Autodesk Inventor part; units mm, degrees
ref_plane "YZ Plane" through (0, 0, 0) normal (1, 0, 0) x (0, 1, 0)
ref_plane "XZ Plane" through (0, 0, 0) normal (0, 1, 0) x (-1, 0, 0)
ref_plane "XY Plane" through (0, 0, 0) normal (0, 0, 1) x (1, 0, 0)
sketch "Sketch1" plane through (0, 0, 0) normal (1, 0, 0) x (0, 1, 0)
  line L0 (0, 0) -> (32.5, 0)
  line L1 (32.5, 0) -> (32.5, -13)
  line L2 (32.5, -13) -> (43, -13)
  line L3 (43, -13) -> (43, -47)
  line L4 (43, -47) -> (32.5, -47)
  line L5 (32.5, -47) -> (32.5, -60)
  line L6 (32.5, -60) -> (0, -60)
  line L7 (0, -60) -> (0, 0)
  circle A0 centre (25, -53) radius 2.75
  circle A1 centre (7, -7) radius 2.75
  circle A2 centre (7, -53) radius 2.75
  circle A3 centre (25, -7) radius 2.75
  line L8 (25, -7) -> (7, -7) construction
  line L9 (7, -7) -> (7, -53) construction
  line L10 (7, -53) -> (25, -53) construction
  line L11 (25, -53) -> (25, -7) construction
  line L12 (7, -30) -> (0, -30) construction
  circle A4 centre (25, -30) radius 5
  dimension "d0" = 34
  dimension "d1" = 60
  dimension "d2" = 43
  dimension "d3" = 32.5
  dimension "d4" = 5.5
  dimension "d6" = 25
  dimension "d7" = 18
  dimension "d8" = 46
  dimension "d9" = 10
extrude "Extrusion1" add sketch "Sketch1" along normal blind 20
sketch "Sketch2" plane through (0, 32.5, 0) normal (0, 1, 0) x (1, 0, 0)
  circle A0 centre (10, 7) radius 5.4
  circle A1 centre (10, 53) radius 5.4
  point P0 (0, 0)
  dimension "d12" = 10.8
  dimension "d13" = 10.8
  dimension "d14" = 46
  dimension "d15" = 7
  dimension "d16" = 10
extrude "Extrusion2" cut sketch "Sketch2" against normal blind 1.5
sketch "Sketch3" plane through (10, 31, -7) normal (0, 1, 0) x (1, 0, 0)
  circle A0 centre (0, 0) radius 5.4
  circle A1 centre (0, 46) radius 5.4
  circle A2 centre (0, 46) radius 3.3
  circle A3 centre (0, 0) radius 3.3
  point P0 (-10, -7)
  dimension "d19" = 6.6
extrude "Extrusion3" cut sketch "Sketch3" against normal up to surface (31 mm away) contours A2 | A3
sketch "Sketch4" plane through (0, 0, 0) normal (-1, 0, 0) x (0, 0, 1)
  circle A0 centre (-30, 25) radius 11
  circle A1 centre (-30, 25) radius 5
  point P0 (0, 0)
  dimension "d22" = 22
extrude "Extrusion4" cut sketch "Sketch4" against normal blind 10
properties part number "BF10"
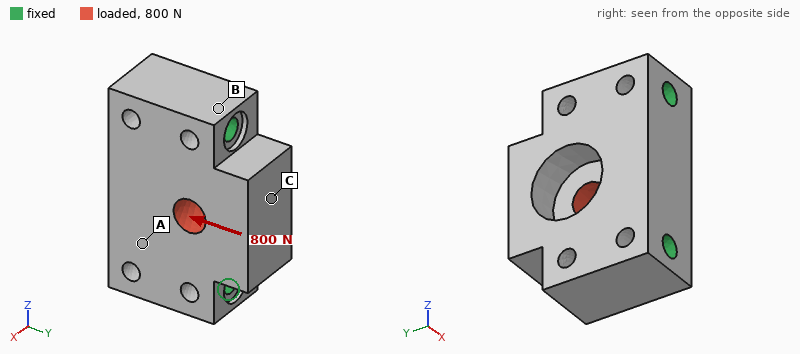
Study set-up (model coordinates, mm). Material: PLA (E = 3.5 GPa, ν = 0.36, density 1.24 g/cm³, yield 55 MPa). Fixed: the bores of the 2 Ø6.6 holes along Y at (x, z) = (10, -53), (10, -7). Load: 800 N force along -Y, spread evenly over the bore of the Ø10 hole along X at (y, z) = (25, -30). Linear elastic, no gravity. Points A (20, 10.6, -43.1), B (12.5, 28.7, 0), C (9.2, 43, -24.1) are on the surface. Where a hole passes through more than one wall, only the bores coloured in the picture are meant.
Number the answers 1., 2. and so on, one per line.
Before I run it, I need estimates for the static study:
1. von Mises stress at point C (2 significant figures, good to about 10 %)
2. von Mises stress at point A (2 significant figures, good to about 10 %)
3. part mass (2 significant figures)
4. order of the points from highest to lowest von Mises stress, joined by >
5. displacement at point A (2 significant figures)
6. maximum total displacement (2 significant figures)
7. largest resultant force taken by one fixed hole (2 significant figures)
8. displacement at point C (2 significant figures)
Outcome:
1. 1.0 MPa
2. 1.8 MPa
3. 47 g
4. A > C > B
5. 8.1 µm
6. 25 µm
7. 410 N
8. 16 µm
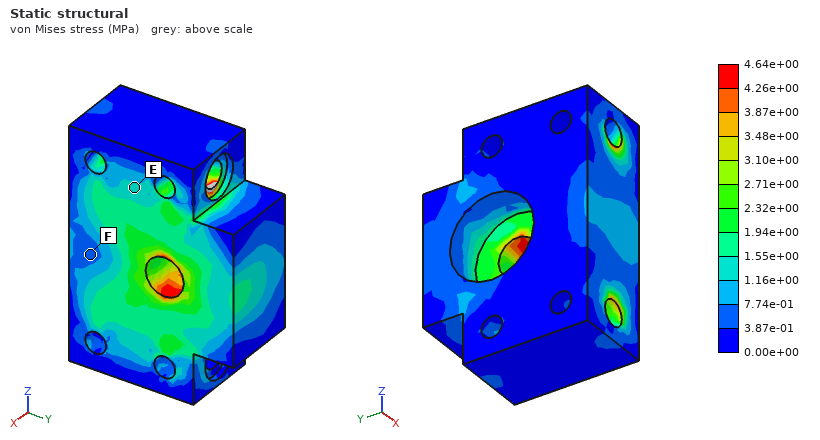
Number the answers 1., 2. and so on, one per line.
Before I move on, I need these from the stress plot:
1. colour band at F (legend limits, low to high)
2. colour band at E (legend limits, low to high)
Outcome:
1. 3.87e-01 to 7.74e-01 MPa
2. 1.16e+00 to 1.55e+00 MPa
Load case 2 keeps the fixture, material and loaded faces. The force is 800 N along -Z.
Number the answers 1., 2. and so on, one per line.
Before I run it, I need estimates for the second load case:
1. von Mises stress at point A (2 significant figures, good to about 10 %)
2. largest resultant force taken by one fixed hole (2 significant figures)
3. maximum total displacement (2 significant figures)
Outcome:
1. 0.53 MPa
2. 410 N
3. 14 µm
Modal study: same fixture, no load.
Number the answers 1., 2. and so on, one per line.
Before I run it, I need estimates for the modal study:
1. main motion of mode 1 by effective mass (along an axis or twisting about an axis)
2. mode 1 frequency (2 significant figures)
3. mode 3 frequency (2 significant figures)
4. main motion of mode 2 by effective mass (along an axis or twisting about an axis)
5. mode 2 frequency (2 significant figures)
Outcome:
1. along X
2. 5200 Hz
3. 9500 Hz
4. along X
5. 8200 Hz
